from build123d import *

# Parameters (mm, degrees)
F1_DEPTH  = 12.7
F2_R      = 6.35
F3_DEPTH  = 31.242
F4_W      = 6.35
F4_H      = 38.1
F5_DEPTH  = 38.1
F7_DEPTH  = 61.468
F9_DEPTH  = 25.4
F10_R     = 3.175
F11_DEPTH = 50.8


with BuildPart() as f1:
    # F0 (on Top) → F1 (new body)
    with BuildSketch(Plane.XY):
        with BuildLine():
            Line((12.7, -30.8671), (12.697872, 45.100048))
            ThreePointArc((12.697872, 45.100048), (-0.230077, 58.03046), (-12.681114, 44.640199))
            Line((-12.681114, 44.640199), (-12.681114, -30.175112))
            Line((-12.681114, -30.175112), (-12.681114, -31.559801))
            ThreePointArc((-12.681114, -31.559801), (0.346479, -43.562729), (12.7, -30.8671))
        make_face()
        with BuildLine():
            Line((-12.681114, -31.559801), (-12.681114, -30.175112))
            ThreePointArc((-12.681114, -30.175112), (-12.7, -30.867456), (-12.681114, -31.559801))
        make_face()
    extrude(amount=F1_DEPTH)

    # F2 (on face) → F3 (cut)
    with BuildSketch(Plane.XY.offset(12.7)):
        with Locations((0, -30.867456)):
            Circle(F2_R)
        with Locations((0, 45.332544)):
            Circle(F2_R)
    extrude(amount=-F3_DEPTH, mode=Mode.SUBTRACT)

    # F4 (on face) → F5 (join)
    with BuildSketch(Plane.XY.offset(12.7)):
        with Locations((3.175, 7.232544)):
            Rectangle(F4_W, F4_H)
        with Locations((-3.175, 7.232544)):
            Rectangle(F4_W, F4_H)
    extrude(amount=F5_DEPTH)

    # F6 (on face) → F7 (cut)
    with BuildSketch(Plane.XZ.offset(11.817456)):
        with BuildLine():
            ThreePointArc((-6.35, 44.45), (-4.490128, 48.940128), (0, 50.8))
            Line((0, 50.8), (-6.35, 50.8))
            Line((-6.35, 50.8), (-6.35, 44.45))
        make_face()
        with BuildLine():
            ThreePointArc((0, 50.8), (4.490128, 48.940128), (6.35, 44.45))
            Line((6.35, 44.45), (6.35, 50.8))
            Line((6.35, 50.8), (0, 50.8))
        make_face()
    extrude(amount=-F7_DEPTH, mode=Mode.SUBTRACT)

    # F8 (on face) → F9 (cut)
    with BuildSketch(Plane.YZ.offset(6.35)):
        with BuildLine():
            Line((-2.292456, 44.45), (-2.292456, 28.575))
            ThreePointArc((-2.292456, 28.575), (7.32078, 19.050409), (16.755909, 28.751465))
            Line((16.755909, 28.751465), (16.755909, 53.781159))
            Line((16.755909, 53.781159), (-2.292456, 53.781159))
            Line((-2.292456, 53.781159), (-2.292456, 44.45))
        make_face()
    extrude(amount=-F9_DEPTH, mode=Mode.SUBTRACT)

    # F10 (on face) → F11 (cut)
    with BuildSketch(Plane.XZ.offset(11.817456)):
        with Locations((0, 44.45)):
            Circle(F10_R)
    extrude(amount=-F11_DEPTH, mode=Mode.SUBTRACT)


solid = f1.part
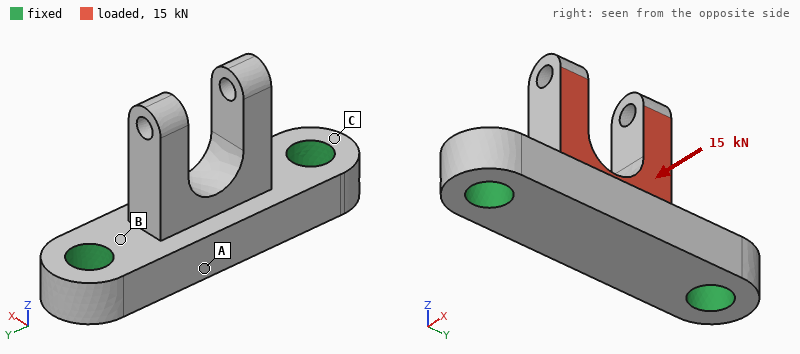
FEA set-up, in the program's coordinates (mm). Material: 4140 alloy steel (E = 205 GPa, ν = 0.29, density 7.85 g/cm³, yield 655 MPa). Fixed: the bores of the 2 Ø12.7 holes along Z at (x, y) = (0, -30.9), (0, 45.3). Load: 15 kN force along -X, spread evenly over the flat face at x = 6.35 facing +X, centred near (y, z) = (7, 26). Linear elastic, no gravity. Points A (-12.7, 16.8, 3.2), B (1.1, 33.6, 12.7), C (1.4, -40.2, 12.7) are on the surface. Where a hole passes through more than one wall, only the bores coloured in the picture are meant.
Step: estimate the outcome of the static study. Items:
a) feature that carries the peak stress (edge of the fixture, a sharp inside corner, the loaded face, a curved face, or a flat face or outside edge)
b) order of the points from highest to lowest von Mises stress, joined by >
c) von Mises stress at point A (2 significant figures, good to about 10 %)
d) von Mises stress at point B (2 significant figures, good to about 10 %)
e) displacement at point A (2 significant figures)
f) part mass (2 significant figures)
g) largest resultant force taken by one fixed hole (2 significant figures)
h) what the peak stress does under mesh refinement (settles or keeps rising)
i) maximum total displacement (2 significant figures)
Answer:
edge of the fixture
B > A > C
79 MPa
250 MPa
0.035 mm
300 g
7.5 kN
keeps rising
0.23 mm
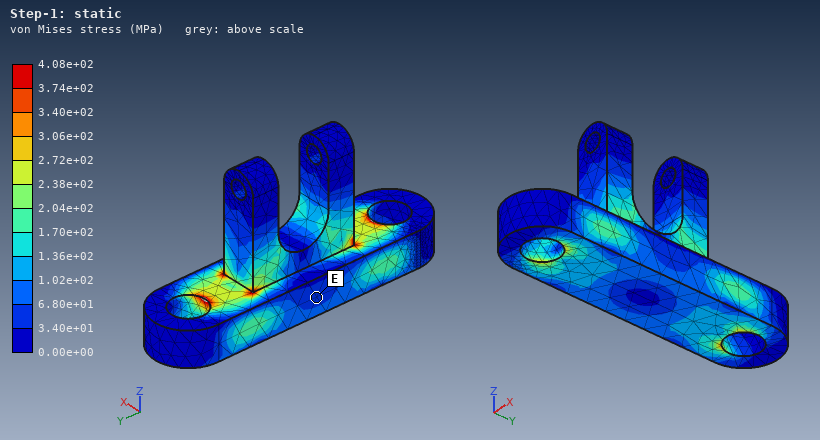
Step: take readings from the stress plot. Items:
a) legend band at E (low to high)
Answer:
3.40e+01 to 6.80e+01 MPa
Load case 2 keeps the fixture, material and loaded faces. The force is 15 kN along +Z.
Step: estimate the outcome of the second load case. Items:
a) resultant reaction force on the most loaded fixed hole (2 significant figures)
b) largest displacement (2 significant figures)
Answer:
7.8 kN
93 µm
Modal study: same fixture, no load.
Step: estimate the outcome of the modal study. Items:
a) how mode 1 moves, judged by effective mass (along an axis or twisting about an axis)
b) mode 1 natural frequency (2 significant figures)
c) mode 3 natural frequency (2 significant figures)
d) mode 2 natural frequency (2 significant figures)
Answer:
along X
5400 Hz
8000 Hz
7500 Hz
